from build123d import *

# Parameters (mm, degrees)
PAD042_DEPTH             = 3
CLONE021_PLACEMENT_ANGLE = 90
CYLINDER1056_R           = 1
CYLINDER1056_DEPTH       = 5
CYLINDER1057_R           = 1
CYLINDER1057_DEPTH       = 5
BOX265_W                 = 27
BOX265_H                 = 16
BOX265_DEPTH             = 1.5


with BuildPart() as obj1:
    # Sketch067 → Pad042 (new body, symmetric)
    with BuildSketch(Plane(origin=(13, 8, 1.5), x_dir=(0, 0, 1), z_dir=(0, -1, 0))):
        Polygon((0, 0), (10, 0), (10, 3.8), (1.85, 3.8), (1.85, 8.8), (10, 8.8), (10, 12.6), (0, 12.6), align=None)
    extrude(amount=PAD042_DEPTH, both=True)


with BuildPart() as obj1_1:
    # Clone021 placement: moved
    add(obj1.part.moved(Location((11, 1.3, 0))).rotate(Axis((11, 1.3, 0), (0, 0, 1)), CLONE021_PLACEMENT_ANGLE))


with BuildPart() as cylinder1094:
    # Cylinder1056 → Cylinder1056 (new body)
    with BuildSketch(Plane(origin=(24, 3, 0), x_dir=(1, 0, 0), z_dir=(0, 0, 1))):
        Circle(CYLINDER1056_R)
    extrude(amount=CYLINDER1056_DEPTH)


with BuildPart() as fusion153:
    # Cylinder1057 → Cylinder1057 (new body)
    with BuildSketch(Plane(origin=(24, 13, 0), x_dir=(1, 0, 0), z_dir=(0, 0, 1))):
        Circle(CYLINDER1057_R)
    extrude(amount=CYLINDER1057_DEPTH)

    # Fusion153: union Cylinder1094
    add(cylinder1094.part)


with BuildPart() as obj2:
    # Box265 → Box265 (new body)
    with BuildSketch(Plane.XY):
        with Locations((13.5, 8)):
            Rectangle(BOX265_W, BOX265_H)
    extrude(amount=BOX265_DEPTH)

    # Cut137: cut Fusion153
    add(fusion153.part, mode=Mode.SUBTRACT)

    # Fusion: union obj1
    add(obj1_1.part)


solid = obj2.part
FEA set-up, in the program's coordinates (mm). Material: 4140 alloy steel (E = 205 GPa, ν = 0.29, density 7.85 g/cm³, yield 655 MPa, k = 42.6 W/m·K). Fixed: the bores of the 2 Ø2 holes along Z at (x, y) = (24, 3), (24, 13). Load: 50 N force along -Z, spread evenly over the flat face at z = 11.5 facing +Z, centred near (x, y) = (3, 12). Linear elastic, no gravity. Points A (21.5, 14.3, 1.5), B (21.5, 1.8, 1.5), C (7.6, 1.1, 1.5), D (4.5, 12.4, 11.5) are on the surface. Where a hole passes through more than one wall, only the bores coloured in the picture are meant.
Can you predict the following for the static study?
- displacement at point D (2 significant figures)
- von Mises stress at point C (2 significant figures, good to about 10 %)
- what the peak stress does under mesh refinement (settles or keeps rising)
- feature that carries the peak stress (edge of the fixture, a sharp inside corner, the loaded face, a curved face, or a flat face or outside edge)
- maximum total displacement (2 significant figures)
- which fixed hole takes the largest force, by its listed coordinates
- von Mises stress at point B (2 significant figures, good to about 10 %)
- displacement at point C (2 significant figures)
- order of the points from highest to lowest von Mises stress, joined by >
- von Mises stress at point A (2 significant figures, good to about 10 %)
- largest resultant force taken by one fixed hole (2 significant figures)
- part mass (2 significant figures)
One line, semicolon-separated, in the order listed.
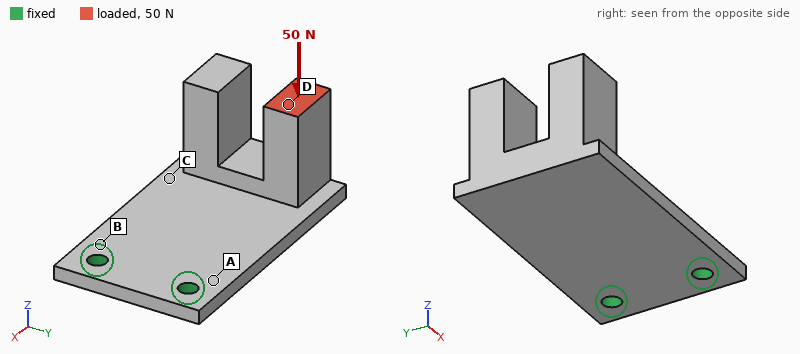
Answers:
0.19 mm; 51 MPa; keeps rising; edge of the fixture; 0.24 mm; (24, 13); 140 MPa; 0.094 mm; A > B > C > D; 180 MPa; 44 N; 9.0 g
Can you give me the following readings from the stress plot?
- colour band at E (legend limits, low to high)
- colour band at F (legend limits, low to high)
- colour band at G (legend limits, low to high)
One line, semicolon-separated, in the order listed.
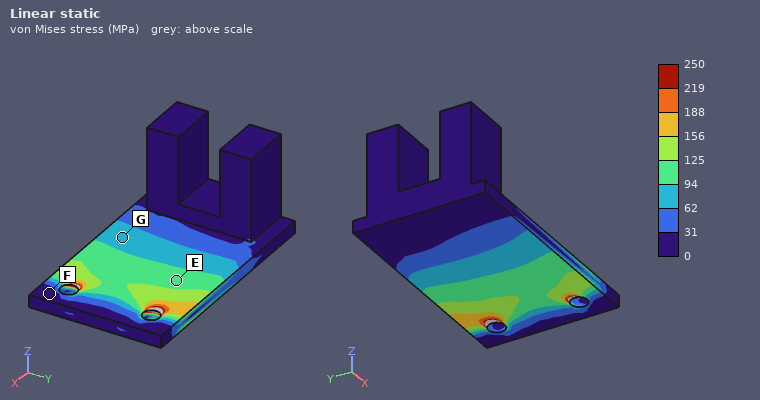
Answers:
94 to 125 MPa; 0 to 31 MPa; 62 to 94 MPa
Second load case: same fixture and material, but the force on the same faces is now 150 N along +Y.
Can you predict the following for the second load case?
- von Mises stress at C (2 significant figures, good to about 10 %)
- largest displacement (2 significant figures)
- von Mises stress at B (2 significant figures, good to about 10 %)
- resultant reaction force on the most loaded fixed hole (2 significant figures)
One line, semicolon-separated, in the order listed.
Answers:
180 MPa; 0.20 mm; 160 MPa; 320 N
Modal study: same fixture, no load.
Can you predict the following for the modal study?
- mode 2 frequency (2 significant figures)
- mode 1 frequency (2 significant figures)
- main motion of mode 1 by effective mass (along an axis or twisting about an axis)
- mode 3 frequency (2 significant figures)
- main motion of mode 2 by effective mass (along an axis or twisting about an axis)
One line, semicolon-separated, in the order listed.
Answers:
3200 Hz; 1100 Hz; along Z; 6100 Hz; along Y
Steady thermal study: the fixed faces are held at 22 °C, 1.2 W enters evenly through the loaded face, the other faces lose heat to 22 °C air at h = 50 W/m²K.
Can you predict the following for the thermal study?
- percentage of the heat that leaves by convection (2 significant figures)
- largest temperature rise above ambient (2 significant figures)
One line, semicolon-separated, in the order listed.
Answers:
51 %; 25 K
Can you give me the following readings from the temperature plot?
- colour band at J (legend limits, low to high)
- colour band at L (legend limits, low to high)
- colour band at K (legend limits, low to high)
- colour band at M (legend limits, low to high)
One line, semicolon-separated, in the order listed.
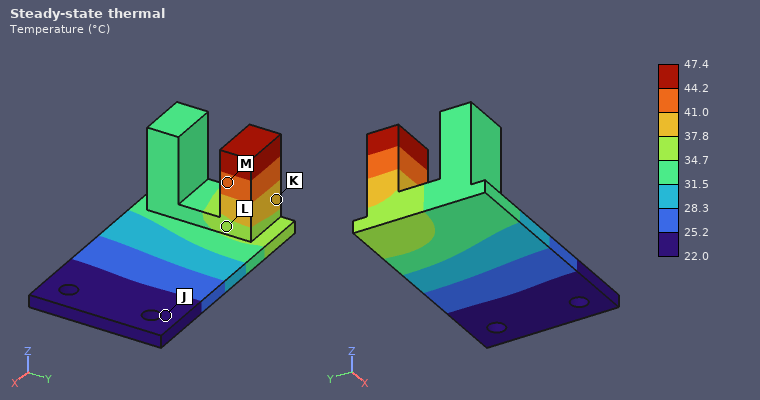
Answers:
22.0 to 25.2 °C; 34.7 to 37.8 °C; 37.8 to 41.0 °C; 41.0 to 44.2 °C
